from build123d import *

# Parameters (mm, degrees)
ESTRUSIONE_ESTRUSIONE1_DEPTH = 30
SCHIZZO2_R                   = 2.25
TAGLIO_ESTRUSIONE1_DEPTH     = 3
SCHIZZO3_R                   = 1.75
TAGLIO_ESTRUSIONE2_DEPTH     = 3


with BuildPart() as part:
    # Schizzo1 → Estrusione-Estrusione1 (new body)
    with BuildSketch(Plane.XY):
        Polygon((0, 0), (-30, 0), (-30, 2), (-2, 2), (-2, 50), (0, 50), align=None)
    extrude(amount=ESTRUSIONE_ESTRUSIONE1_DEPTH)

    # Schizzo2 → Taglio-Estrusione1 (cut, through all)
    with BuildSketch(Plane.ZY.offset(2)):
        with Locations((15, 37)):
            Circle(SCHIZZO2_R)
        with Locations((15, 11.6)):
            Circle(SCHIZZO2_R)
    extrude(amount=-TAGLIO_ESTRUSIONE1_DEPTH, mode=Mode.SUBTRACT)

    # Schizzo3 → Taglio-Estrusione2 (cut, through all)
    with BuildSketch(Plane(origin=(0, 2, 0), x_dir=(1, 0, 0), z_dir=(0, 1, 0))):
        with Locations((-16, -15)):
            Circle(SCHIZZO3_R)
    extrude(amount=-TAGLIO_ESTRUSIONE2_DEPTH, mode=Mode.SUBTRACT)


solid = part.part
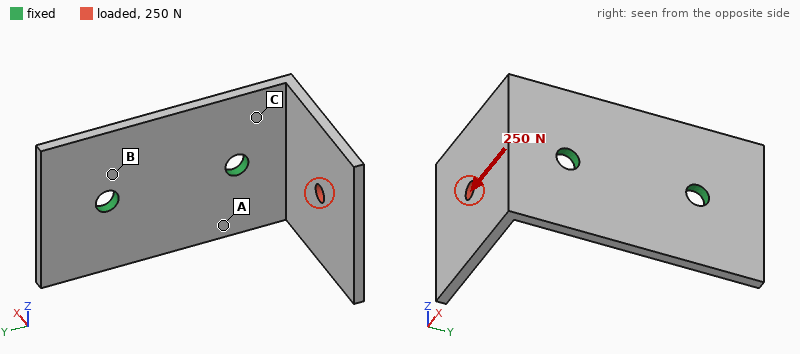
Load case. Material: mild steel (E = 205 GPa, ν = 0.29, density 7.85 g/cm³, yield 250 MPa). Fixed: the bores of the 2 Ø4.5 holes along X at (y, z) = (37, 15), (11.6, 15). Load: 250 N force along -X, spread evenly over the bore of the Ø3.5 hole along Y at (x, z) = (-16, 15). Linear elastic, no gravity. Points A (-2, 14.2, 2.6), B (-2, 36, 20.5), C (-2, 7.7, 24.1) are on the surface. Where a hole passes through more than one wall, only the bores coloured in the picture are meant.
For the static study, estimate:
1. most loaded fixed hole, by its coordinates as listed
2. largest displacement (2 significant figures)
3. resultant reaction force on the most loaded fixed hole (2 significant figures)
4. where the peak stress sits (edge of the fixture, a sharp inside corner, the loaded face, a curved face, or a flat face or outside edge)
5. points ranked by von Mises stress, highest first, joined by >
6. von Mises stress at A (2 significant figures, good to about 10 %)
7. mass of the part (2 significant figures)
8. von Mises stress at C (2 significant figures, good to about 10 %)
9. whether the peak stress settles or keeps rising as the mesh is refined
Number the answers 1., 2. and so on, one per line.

1. (11.6, 15)
2. 0.10 mm
3. 270 N
4. edge of the fixture
5. C > A > B
6. 32 MPa
7. 36 g
8. 55 MPa
9. keeps rising
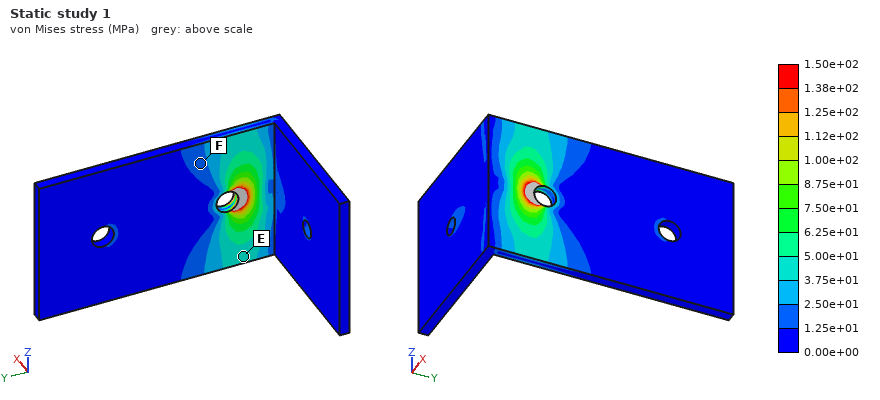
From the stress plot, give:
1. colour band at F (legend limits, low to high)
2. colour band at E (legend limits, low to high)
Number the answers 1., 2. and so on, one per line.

1. 1.25e+01 to 2.50e+01 MPa
2. 3.75e+01 to 5.00e+01 MPa
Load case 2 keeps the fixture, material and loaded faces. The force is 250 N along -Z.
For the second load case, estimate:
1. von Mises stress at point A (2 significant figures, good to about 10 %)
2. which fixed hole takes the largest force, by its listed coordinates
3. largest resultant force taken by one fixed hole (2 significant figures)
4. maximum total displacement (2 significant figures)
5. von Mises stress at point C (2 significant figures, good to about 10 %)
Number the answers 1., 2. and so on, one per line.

1. 68 MPa
2. (11.6, 15)
3. 330 N
4. 0.16 mm
5. 59 MPa
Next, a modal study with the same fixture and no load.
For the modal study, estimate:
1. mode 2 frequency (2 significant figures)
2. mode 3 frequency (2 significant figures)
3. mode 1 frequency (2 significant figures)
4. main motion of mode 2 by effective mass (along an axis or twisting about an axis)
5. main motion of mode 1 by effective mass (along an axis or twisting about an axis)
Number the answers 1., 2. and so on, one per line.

1. 2000 Hz
2. 4300 Hz
3. 1300 Hz
4. along Z
5. along Y
